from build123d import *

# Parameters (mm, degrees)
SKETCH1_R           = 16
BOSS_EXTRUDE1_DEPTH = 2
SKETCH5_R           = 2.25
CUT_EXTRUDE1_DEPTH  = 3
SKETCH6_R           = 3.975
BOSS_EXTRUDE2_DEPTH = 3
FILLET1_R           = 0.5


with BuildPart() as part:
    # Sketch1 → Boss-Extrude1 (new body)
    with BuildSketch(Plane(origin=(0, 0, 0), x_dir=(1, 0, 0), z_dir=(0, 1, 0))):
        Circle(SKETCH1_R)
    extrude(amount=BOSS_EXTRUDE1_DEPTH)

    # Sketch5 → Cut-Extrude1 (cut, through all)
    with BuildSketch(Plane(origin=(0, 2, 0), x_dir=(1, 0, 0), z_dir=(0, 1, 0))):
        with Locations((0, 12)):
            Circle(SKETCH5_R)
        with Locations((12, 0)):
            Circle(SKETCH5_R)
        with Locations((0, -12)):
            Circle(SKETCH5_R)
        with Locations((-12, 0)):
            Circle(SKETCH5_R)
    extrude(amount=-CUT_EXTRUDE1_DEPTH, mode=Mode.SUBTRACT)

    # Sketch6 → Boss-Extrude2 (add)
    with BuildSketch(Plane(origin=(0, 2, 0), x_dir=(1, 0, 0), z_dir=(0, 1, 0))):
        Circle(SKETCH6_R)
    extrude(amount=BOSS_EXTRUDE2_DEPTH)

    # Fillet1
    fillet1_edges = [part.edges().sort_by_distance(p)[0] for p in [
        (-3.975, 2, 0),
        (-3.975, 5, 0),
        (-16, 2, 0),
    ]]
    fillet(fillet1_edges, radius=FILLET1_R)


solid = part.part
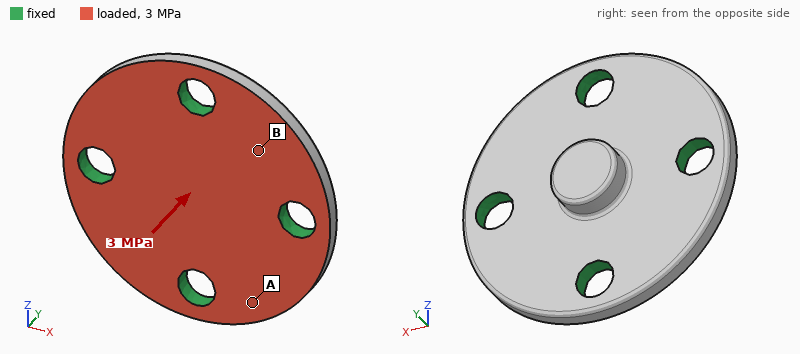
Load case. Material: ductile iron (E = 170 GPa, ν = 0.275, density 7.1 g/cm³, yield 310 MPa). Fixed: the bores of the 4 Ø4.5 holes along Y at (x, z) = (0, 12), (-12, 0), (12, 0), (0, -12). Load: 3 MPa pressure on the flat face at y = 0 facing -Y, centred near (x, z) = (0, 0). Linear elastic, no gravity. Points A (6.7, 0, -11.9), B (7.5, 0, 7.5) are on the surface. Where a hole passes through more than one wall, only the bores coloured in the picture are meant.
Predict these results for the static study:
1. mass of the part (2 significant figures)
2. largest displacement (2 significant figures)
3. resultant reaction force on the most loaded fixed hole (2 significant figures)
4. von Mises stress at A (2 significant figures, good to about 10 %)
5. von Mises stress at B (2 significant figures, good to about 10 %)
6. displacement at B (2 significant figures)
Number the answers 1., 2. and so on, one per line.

1. 12 g
2. 8.7 µm
3. 560 N
4. 21 MPa
5. 49 MPa
6. 4.4 µm
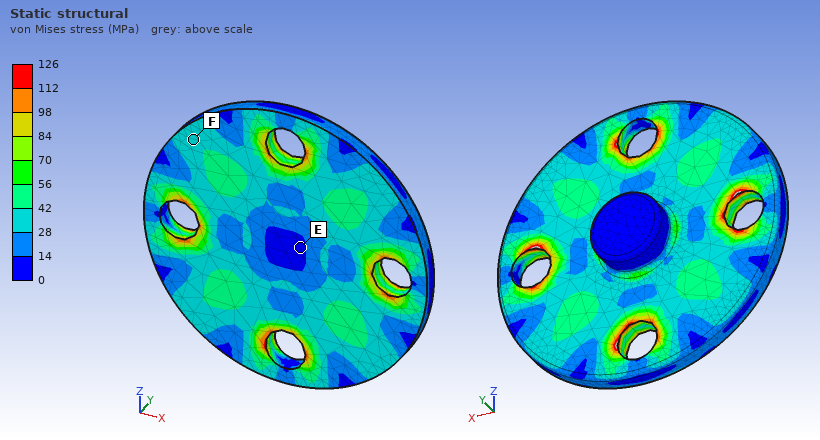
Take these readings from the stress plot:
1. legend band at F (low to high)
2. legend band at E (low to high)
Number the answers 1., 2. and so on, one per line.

1. 28 to 42 MPa
2. 0 to 14 MPa
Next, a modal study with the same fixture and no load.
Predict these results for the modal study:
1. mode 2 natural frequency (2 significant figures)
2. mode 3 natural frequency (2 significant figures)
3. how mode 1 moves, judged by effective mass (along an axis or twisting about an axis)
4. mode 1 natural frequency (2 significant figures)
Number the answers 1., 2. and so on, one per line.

1. 32 kHz
2. 32 kHz
3. along Y
4. 30 kHz
